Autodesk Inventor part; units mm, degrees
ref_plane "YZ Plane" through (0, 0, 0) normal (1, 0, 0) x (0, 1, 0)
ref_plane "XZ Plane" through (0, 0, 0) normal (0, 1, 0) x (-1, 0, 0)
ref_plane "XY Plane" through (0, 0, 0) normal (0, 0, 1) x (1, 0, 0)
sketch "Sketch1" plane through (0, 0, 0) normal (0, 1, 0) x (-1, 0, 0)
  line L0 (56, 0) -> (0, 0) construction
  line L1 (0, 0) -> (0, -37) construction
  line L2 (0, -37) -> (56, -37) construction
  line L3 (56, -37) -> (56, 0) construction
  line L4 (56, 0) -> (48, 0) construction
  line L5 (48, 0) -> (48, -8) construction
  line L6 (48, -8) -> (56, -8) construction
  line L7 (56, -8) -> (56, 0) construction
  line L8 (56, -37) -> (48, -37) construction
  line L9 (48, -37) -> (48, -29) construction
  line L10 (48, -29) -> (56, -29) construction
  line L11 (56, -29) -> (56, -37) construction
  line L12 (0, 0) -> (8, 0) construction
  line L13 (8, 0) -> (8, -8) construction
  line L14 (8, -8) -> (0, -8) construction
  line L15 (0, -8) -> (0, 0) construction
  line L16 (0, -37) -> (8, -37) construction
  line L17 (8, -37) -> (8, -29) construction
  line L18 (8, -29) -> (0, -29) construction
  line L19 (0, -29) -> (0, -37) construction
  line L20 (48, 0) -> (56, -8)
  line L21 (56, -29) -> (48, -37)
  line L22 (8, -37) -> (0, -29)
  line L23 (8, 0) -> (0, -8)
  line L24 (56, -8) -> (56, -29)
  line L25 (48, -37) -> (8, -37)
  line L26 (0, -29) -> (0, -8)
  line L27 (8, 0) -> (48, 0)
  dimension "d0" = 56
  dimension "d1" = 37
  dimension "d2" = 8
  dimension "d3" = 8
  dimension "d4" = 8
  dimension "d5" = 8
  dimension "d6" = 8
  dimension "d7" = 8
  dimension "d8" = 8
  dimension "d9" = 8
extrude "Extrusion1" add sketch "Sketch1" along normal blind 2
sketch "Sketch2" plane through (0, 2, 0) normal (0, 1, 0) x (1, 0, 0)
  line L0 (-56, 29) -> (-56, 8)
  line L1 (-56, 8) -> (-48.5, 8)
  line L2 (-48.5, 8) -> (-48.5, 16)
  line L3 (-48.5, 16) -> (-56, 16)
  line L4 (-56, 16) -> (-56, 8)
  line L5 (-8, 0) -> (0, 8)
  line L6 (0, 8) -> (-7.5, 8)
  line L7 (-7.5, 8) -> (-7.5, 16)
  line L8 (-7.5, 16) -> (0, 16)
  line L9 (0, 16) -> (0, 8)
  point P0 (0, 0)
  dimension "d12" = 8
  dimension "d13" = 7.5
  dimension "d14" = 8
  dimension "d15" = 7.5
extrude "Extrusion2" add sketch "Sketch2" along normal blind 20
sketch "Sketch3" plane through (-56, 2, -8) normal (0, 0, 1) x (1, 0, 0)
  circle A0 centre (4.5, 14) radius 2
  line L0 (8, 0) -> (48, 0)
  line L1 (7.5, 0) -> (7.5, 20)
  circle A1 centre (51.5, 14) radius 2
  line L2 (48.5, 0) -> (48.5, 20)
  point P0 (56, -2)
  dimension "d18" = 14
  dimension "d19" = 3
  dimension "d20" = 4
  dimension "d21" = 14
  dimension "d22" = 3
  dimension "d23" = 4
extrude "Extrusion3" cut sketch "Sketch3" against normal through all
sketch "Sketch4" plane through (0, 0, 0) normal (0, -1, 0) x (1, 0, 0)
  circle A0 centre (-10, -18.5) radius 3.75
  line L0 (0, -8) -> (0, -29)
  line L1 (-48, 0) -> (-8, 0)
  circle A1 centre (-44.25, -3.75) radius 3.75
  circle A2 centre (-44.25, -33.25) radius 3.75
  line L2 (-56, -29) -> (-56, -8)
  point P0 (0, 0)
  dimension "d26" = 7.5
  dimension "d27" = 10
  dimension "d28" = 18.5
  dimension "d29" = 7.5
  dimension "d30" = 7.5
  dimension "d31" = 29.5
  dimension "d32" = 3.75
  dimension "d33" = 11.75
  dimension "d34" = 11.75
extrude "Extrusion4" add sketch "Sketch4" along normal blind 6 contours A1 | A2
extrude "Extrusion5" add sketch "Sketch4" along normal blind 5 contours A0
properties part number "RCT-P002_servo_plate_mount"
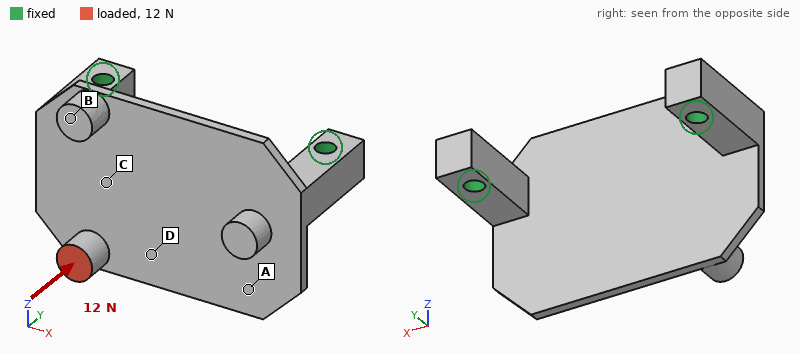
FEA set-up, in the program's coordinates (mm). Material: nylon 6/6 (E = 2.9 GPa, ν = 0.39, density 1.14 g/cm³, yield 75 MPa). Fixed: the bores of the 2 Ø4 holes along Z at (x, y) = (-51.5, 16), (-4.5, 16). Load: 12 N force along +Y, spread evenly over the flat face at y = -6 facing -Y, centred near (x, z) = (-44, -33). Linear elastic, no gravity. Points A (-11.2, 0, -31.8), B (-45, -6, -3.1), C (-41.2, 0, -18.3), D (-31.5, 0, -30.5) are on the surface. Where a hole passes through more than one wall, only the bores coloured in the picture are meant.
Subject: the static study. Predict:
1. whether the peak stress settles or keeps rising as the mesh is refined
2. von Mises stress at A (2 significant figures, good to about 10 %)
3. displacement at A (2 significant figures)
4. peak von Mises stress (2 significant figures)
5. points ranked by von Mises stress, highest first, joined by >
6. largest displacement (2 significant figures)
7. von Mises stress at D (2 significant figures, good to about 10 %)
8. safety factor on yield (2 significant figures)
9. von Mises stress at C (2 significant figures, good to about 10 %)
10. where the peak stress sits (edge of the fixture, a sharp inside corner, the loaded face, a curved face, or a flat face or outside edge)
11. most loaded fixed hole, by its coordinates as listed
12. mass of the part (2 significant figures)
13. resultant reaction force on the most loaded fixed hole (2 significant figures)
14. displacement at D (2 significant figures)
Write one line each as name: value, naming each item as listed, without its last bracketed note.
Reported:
whether the peak stress settles or keeps rising as the mesh is refined: settles
von Mises stress at A: 1.9 MPa
displacement at A: 0.19 mm
peak von Mises stress: 14 MPa
points ranked by von Mises stress, highest first, joined by >: C > D > A > B
largest displacement: 0.74 mm
von Mises stress at D: 3.7 MPa
safety factor on yield: 5.4
von Mises stress at C: 5.3 MPa
where the peak stress sits: a flat face or outside edge
most loaded fixed hole, by its coordinates as listed: (-51.5, 16)
mass of the part: 7.8 g
resultant reaction force on the most loaded fixed hole: 11 N
displacement at D: 0.39 mm
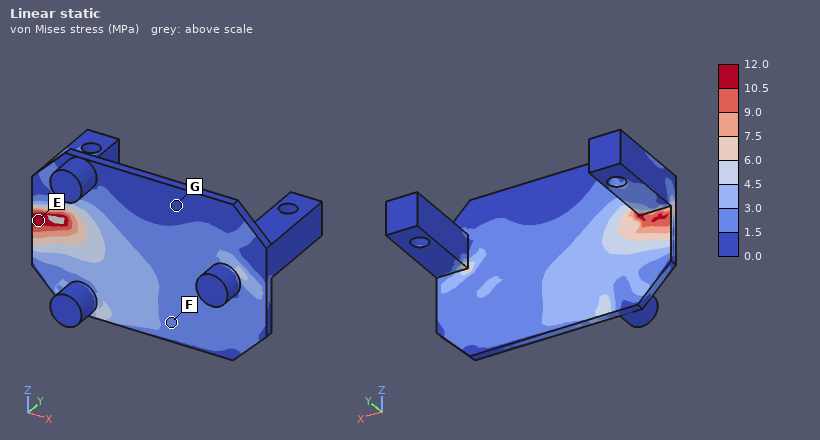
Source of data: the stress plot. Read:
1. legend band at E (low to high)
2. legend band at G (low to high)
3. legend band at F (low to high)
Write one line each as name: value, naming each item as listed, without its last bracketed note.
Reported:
legend band at E: 10.5 to 12.0 MPa
legend band at G: 0.0 to 1.5 MPa
legend band at F: 1.5 to 3.0 MPa
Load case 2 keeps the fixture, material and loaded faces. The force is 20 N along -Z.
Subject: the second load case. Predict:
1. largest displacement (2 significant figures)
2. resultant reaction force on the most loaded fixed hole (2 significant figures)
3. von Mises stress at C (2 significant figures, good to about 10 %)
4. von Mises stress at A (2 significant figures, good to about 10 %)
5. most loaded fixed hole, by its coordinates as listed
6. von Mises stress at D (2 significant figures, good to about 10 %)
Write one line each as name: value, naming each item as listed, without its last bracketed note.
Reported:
largest displacement: 0.71 mm
resultant reaction force on the most loaded fixed hole: 16 N
von Mises stress at C: 4.4 MPa
von Mises stress at A: 1.7 MPa
most loaded fixed hole, by its coordinates as listed: (-51.5, 16)
von Mises stress at D: 4.6 MPa
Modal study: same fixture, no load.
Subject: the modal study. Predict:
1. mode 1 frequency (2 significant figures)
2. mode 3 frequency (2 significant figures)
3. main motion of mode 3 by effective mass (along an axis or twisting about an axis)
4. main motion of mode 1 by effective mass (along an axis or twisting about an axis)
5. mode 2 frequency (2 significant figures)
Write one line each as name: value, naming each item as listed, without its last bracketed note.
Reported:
mode 1 frequency: 690 Hz
mode 3 frequency: 1500 Hz
main motion of mode 3 by effective mass: along Y
main motion of mode 1 by effective mass: along Y
mode 2 frequency: 1400 Hz
